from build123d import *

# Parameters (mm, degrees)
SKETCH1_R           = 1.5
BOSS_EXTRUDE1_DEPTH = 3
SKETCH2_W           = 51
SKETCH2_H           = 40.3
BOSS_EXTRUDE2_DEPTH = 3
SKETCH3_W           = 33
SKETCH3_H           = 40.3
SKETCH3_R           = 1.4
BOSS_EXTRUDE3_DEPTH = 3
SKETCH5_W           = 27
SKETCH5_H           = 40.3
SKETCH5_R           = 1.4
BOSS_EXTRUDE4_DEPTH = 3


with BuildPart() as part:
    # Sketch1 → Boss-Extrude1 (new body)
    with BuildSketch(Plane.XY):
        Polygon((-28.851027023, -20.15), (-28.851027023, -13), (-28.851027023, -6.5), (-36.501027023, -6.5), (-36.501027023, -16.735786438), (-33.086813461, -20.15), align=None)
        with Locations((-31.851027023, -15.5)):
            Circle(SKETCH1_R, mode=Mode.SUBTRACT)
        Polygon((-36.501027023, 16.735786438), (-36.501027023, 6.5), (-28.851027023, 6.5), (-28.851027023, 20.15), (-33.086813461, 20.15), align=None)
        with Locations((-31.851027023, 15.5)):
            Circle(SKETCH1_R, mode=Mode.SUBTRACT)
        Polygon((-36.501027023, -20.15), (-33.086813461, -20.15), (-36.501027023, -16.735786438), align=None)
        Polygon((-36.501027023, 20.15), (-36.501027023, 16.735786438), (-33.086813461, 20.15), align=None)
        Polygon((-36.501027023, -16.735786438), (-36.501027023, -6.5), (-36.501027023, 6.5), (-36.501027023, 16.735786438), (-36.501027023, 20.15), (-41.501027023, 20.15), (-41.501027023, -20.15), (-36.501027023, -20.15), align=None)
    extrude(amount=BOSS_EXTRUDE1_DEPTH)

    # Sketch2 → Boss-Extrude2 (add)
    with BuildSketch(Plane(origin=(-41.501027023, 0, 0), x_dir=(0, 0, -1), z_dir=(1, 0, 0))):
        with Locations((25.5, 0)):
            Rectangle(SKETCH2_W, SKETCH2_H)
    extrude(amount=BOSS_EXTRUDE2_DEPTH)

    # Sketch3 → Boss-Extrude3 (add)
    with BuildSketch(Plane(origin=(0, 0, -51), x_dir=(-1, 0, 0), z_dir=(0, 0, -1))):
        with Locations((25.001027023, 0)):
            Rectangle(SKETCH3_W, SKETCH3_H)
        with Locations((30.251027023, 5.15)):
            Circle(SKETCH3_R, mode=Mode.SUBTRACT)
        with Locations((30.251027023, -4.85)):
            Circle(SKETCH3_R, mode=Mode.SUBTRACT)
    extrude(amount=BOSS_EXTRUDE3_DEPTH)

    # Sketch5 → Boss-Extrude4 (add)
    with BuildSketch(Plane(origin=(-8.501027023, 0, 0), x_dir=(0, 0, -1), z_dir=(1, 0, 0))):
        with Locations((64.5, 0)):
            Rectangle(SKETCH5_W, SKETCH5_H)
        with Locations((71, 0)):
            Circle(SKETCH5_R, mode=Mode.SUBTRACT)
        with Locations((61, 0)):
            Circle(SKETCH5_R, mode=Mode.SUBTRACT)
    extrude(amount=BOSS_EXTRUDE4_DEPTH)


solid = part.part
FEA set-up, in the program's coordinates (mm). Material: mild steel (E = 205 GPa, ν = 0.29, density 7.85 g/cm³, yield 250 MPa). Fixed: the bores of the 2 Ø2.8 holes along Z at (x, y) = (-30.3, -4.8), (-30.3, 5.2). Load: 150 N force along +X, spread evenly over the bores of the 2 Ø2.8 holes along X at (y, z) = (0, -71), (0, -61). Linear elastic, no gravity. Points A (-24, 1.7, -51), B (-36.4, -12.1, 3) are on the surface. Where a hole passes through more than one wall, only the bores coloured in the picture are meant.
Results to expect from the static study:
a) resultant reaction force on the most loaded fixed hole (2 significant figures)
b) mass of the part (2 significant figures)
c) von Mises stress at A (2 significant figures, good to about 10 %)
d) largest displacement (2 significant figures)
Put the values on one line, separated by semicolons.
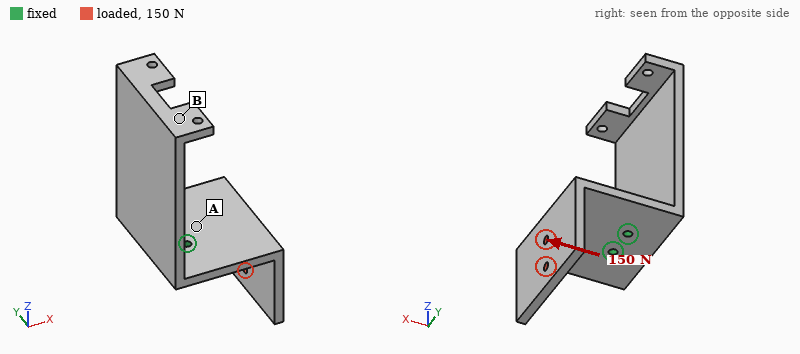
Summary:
79 N; 110 g; 32 MPa; 87 µm
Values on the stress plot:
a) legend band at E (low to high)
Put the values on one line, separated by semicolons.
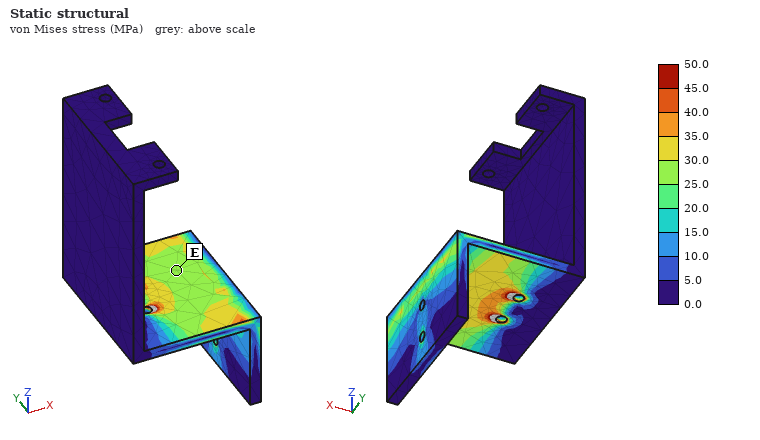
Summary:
25.0 to 30.0 MPa
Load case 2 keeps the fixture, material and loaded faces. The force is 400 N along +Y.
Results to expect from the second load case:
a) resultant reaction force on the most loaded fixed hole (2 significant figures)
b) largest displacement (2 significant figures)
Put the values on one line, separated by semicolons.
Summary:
860 N; 100 µm
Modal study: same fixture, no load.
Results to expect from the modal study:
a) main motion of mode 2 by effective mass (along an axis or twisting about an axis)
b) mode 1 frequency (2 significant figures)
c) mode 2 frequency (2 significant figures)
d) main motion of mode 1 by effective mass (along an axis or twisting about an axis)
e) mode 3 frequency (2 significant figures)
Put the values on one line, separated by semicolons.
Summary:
along Y; 520 Hz; 1300 Hz; along X; 1400 Hz
